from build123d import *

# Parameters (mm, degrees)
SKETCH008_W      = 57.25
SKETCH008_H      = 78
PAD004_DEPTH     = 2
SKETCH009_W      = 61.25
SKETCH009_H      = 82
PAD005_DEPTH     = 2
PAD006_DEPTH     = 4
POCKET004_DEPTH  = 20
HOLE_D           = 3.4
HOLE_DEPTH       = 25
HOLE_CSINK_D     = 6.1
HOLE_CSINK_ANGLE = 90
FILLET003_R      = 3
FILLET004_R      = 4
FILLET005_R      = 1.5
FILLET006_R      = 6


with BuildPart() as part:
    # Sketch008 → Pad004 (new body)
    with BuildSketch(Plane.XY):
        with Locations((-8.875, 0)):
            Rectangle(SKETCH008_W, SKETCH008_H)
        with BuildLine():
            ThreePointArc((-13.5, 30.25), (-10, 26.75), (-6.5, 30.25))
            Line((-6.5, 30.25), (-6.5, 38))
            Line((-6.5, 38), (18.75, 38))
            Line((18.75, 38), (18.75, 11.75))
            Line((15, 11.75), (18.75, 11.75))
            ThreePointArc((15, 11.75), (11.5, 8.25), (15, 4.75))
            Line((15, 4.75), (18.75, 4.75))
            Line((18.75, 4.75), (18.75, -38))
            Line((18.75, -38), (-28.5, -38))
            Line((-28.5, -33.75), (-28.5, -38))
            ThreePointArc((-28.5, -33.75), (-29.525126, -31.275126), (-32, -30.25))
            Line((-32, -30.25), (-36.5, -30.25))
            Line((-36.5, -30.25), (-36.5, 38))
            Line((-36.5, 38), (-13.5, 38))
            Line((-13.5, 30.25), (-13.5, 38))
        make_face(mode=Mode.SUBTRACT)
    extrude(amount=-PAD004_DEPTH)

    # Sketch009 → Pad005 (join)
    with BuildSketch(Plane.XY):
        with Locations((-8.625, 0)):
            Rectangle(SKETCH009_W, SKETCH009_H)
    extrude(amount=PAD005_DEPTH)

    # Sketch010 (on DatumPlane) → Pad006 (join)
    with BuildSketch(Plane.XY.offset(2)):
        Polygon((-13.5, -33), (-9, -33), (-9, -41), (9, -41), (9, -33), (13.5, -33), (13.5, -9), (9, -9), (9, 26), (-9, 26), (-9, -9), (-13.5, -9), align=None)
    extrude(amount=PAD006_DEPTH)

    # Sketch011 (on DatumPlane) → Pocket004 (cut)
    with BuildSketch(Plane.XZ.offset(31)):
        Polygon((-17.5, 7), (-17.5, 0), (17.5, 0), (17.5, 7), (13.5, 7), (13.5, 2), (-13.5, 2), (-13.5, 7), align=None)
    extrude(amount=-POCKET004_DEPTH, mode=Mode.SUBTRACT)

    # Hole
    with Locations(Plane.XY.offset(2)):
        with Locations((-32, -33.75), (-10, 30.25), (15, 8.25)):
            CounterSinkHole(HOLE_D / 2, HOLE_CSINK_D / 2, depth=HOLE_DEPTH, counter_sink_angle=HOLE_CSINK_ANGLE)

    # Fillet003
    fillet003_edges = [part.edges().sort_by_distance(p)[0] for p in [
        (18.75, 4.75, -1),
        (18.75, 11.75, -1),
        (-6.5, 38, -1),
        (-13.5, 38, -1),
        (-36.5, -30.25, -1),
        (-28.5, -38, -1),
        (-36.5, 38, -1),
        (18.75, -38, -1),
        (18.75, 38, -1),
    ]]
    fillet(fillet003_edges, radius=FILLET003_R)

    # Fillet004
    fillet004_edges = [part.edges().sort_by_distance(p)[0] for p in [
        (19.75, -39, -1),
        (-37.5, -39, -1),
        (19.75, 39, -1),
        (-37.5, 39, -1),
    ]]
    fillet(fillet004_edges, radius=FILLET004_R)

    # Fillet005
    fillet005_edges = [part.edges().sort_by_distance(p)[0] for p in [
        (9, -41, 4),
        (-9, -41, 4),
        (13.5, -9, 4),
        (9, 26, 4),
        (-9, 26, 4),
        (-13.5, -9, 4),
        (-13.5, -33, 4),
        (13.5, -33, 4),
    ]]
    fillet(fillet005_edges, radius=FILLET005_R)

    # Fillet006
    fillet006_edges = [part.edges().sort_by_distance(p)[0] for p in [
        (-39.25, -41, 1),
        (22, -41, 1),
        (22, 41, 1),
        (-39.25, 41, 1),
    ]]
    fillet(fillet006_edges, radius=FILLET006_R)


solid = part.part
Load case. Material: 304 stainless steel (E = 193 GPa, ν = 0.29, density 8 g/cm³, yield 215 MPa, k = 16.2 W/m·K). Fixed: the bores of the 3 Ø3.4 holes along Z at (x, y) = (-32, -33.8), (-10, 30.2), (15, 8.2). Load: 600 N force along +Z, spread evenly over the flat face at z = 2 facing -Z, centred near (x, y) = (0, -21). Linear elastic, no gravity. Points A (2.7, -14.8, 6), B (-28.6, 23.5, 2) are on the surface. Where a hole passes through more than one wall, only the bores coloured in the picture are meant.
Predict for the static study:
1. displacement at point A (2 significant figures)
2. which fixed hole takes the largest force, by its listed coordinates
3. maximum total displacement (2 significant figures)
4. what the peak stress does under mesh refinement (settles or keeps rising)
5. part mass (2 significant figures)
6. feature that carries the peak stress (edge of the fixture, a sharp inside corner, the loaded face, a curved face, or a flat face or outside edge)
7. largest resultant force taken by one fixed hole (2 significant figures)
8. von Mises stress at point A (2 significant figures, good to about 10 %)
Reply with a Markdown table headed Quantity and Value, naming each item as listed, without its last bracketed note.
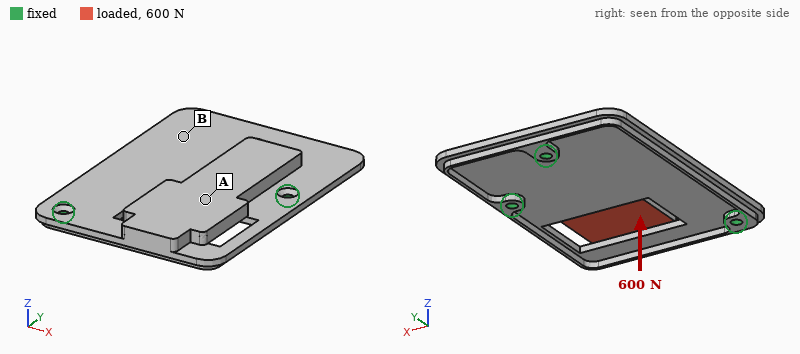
| Quantity | Value |
|---|---|
| displacement at point A | 0.054 mm |
| which fixed hole takes the largest force, by its listed coordinates | (15, 8.2) |
| maximum total displacement | 0.11 mm |
| what the peak stress does under mesh refinement | keeps rising |
| part mass | 120 g |
| feature that carries the peak stress | a sharp inside corner |
| largest resultant force taken by one fixed hole | 950 N |
| von Mises stress at point A | 37 MPa |
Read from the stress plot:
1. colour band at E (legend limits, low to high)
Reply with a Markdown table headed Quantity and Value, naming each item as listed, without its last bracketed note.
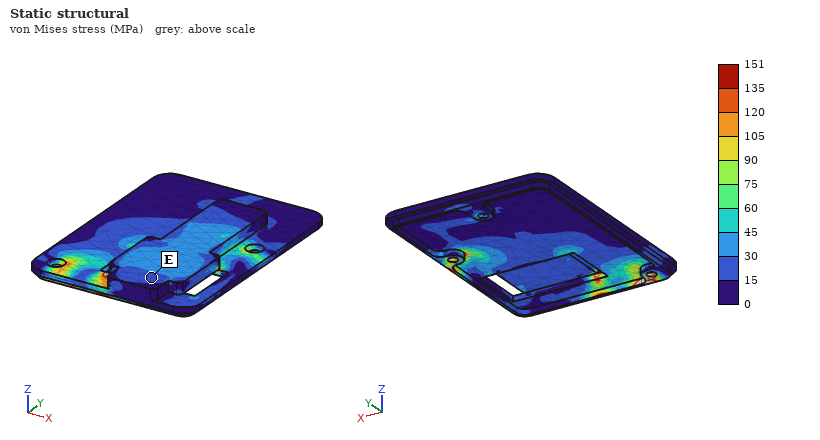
| Quantity | Value |
|---|---|
| colour band at E | 15 to 30 MPa |
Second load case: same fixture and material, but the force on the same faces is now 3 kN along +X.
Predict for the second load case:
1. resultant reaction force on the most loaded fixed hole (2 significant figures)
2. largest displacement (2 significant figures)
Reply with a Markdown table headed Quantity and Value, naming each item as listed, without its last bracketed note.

| Quantity | Value |
|---|---|
| resultant reaction force on the most loaded fixed hole | 1.6 kN |
| largest displacement | 17 µm |
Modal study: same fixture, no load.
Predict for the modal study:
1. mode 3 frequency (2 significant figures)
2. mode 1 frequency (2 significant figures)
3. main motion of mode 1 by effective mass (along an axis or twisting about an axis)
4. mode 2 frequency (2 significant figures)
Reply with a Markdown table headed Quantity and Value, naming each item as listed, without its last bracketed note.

| Quantity | Value |
|---|---|
| mode 3 frequency | 3800 Hz |
| mode 1 frequency | 2100 Hz |
| main motion of mode 1 by effective mass | along Z |
| mode 2 frequency | 2200 Hz |
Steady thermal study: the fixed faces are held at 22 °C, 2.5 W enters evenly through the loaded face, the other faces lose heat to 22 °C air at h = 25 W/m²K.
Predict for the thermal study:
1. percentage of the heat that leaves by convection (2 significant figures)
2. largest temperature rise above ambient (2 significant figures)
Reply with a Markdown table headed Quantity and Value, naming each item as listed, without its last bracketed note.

| Quantity | Value |
|---|---|
| percentage of the heat that leaves by convection | 63 % |
| largest temperature rise above ambient | 19 K |
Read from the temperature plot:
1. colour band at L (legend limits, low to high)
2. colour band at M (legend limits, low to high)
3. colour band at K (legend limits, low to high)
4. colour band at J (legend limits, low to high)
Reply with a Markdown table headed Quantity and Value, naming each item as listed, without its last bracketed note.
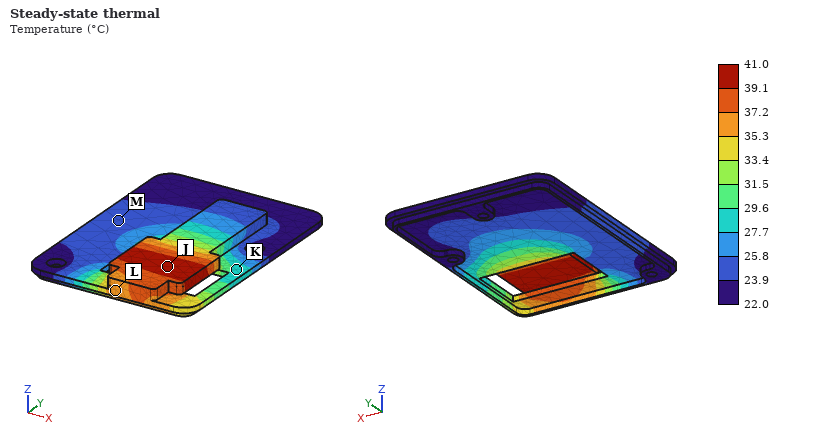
| Quantity | Value |
|---|---|
| colour band at L | 35.3 to 37.2 °C |
| colour band at M | 23.9 to 25.8 °C |
| colour band at K | 27.7 to 29.6 °C |
| colour band at J | 39.1 to 41.0 °C |
